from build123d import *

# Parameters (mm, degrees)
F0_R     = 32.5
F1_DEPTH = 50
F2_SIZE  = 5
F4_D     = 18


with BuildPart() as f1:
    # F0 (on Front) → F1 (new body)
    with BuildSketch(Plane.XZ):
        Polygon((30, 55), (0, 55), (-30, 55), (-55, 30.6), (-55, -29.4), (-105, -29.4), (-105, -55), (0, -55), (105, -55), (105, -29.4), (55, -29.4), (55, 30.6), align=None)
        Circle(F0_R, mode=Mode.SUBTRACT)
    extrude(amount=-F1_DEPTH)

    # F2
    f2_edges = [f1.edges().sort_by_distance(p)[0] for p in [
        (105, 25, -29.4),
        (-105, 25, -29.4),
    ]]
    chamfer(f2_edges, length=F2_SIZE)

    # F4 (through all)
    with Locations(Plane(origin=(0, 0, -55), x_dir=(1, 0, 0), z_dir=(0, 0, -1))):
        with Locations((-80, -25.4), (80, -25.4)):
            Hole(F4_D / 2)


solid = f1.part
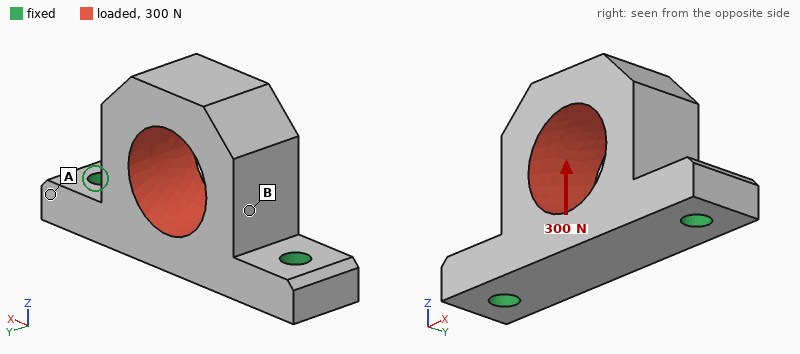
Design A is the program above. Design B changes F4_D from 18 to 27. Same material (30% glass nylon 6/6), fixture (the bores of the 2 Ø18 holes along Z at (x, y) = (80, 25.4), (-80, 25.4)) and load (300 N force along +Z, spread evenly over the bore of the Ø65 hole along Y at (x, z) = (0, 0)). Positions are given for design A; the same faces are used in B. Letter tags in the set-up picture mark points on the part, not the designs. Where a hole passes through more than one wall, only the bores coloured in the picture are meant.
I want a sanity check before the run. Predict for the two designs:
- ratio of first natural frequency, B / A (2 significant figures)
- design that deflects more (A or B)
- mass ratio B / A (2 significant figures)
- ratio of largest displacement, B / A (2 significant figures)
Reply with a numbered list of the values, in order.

1. 1.1
2. A
3. 0.97
4. 0.77
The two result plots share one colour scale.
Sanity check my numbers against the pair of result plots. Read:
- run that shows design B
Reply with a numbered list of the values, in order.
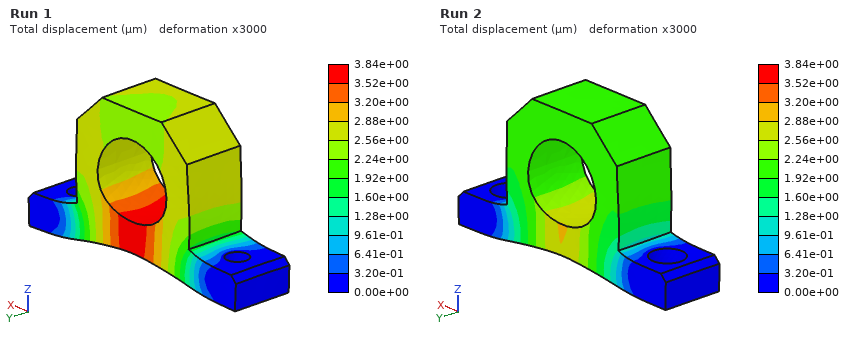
1. Run 2
